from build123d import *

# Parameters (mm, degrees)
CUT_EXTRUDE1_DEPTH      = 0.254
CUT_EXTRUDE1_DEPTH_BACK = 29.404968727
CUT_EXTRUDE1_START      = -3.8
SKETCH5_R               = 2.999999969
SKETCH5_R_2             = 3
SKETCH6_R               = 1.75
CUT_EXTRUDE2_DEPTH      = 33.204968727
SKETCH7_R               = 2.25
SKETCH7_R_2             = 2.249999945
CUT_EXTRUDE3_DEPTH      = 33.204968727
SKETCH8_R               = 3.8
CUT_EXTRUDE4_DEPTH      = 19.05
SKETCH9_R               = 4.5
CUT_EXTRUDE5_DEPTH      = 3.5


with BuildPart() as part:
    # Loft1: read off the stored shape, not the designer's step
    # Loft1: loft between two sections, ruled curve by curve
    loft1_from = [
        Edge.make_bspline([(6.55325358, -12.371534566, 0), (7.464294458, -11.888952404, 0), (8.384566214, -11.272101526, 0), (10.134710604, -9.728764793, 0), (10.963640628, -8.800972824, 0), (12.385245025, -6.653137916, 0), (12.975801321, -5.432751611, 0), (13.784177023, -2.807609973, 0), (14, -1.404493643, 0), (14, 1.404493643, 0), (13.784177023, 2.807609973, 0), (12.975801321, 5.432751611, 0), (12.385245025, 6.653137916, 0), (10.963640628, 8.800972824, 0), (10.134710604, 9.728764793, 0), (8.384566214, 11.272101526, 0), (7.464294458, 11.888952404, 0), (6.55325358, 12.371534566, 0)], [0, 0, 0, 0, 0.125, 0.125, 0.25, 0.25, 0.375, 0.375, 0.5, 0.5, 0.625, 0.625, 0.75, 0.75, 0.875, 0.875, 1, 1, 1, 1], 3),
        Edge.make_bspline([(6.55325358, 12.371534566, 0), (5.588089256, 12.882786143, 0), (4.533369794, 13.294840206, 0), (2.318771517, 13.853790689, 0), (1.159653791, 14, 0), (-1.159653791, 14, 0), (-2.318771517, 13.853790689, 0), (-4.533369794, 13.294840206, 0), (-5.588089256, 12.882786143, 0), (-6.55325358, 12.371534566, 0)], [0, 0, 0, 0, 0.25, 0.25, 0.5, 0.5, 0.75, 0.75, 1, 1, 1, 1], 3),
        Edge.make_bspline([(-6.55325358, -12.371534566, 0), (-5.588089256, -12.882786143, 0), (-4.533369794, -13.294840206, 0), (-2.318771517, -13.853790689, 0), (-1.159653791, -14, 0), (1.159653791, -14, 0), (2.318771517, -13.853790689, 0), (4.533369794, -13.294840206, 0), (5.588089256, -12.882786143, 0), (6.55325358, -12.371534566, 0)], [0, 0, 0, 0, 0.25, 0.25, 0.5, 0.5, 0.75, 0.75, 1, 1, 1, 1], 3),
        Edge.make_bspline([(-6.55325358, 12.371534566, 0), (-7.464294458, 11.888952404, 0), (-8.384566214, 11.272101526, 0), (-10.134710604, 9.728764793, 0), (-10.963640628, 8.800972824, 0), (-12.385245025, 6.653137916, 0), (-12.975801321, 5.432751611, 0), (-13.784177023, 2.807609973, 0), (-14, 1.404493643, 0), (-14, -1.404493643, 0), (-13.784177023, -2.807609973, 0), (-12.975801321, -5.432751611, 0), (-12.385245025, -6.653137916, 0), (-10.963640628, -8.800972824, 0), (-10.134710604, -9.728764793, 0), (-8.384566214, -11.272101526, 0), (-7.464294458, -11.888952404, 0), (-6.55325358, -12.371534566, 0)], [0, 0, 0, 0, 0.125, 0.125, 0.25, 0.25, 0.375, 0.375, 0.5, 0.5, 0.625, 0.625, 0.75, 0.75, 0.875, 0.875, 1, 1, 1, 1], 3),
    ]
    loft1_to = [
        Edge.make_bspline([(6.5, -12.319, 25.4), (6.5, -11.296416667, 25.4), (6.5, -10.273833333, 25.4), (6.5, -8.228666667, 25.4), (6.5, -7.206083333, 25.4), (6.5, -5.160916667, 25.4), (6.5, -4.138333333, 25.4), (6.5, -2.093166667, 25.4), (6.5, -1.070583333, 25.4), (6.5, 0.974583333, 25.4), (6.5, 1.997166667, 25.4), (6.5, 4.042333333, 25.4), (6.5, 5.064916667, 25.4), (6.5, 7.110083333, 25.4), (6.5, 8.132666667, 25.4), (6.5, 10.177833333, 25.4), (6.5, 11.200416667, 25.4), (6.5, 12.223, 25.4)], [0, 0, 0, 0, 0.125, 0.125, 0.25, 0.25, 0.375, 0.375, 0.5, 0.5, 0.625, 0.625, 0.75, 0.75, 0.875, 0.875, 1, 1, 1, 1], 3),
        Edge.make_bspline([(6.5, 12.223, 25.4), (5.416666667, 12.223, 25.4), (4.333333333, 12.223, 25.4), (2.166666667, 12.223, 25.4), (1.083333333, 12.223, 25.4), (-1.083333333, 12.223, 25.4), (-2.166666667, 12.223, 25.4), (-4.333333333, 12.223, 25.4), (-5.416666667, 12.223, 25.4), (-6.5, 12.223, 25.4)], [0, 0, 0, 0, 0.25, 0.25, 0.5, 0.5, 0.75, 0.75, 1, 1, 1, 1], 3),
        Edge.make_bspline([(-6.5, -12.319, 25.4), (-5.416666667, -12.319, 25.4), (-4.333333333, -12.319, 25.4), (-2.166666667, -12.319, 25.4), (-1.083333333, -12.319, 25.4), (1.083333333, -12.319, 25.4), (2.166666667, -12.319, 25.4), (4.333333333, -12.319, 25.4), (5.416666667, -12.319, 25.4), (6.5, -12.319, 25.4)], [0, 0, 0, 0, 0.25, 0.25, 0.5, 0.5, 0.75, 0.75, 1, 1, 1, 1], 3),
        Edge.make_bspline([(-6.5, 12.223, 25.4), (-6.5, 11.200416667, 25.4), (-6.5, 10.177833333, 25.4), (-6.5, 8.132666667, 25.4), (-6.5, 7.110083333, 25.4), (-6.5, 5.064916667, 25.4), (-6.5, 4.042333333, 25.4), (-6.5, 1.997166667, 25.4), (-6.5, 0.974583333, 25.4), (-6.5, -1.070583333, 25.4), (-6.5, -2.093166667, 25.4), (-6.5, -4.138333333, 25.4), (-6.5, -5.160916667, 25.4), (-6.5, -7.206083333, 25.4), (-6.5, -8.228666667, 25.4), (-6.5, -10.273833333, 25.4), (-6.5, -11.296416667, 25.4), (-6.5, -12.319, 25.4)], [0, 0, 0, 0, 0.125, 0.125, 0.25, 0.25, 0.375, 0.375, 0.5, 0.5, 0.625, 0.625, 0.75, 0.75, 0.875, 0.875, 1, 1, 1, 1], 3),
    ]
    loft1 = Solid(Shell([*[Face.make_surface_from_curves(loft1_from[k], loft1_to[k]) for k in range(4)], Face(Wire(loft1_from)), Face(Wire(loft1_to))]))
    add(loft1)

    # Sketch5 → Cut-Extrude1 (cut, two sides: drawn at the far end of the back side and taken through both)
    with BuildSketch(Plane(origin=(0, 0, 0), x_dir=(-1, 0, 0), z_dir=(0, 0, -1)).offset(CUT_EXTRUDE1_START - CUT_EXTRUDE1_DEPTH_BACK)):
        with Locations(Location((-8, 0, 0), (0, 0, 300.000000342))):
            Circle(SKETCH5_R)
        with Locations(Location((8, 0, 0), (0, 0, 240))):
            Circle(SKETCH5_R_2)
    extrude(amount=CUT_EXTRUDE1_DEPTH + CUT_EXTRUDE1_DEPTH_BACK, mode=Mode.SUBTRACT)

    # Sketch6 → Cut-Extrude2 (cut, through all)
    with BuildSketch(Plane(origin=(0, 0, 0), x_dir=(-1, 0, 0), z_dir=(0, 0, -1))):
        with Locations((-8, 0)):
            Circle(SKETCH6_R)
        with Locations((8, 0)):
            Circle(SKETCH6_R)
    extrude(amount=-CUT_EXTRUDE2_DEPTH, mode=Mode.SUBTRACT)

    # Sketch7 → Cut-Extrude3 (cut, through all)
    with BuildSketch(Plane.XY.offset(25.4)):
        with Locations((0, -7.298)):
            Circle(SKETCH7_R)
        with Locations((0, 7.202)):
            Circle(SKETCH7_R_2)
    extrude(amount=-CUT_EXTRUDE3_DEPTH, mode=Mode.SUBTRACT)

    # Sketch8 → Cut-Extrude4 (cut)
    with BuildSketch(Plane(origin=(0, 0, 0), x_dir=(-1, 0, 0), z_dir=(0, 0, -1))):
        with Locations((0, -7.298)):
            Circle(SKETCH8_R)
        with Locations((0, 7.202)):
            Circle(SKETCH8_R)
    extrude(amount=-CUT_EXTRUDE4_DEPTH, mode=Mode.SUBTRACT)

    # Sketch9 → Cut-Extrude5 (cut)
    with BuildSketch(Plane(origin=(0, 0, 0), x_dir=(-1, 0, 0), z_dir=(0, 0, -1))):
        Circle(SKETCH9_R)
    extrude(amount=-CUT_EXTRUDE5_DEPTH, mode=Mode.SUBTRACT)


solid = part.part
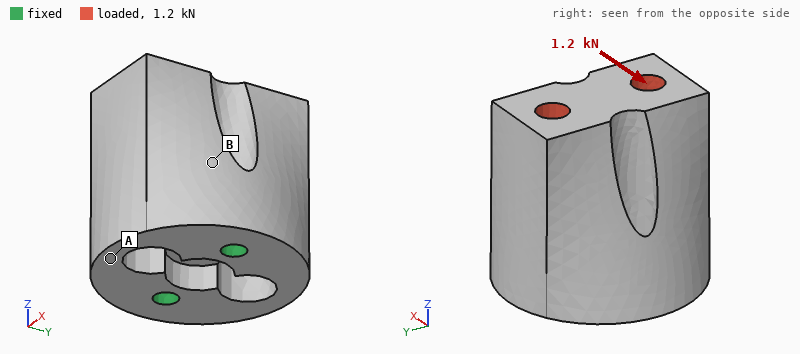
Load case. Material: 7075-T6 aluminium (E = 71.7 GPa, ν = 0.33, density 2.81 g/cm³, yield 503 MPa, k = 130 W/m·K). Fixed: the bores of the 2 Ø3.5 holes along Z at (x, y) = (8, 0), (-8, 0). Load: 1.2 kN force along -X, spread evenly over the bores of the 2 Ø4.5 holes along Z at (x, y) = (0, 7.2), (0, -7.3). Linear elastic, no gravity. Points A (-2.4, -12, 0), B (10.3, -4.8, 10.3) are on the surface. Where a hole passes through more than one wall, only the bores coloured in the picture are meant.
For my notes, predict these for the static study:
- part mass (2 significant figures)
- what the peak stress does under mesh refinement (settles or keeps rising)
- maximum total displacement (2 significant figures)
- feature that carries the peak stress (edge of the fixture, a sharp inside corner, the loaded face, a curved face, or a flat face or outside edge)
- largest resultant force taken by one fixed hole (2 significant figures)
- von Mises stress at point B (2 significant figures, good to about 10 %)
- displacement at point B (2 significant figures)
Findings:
24 g
keeps rising
19 µm
edge of the fixture
1.5 kN
19 MPa
8.4 µm
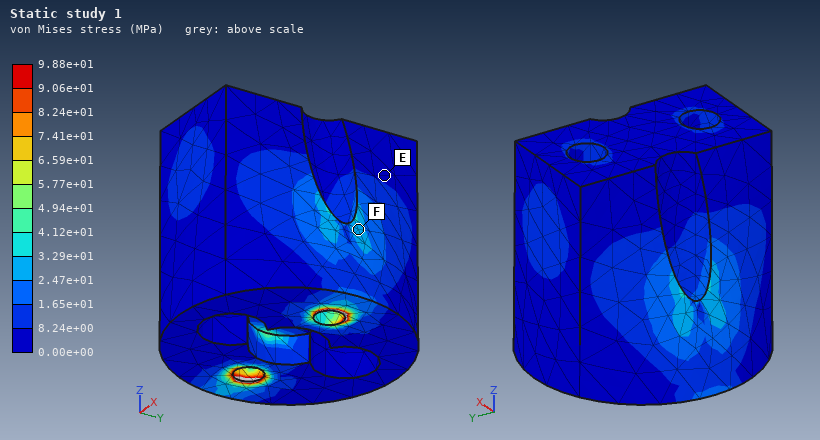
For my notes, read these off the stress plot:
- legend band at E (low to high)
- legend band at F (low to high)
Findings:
0.00e+00 to 8.24e+00 MPa
2.47e+01 to 3.29e+01 MPa
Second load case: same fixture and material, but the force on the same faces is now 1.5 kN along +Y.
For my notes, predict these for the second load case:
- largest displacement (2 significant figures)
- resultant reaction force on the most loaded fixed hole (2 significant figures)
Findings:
0.15 mm
750 N
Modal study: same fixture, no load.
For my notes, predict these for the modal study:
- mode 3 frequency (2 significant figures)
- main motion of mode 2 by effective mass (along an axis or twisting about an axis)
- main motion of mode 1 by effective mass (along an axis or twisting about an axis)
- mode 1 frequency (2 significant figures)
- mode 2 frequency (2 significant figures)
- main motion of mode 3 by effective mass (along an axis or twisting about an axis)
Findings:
23 kHz
along X
along Y
5300 Hz
14 kHz
twisting about Z
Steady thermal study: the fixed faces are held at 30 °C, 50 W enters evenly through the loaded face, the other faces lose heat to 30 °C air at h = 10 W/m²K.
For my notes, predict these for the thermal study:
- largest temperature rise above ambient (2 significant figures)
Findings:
40 K
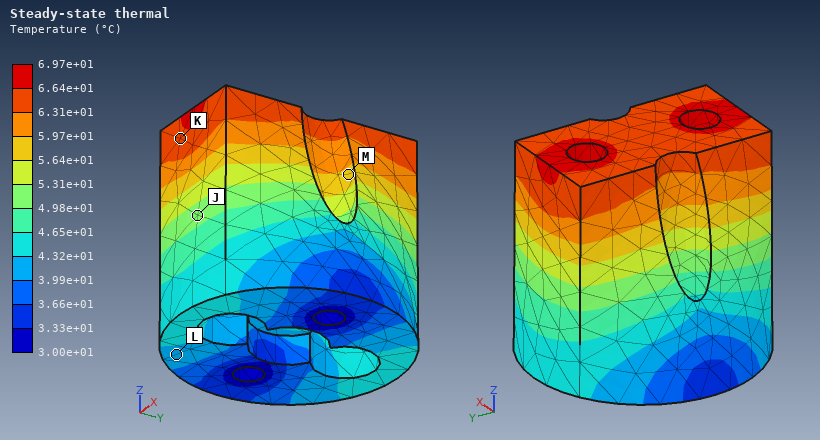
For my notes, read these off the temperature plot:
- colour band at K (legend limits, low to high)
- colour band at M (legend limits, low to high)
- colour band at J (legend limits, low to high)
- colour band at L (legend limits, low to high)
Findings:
6.31e+01 to 6.64e+01 °C
5.64e+01 to 5.97e+01 °C
4.98e+01 to 5.31e+01 °C
3.99e+01 to 4.32e+01 °C
